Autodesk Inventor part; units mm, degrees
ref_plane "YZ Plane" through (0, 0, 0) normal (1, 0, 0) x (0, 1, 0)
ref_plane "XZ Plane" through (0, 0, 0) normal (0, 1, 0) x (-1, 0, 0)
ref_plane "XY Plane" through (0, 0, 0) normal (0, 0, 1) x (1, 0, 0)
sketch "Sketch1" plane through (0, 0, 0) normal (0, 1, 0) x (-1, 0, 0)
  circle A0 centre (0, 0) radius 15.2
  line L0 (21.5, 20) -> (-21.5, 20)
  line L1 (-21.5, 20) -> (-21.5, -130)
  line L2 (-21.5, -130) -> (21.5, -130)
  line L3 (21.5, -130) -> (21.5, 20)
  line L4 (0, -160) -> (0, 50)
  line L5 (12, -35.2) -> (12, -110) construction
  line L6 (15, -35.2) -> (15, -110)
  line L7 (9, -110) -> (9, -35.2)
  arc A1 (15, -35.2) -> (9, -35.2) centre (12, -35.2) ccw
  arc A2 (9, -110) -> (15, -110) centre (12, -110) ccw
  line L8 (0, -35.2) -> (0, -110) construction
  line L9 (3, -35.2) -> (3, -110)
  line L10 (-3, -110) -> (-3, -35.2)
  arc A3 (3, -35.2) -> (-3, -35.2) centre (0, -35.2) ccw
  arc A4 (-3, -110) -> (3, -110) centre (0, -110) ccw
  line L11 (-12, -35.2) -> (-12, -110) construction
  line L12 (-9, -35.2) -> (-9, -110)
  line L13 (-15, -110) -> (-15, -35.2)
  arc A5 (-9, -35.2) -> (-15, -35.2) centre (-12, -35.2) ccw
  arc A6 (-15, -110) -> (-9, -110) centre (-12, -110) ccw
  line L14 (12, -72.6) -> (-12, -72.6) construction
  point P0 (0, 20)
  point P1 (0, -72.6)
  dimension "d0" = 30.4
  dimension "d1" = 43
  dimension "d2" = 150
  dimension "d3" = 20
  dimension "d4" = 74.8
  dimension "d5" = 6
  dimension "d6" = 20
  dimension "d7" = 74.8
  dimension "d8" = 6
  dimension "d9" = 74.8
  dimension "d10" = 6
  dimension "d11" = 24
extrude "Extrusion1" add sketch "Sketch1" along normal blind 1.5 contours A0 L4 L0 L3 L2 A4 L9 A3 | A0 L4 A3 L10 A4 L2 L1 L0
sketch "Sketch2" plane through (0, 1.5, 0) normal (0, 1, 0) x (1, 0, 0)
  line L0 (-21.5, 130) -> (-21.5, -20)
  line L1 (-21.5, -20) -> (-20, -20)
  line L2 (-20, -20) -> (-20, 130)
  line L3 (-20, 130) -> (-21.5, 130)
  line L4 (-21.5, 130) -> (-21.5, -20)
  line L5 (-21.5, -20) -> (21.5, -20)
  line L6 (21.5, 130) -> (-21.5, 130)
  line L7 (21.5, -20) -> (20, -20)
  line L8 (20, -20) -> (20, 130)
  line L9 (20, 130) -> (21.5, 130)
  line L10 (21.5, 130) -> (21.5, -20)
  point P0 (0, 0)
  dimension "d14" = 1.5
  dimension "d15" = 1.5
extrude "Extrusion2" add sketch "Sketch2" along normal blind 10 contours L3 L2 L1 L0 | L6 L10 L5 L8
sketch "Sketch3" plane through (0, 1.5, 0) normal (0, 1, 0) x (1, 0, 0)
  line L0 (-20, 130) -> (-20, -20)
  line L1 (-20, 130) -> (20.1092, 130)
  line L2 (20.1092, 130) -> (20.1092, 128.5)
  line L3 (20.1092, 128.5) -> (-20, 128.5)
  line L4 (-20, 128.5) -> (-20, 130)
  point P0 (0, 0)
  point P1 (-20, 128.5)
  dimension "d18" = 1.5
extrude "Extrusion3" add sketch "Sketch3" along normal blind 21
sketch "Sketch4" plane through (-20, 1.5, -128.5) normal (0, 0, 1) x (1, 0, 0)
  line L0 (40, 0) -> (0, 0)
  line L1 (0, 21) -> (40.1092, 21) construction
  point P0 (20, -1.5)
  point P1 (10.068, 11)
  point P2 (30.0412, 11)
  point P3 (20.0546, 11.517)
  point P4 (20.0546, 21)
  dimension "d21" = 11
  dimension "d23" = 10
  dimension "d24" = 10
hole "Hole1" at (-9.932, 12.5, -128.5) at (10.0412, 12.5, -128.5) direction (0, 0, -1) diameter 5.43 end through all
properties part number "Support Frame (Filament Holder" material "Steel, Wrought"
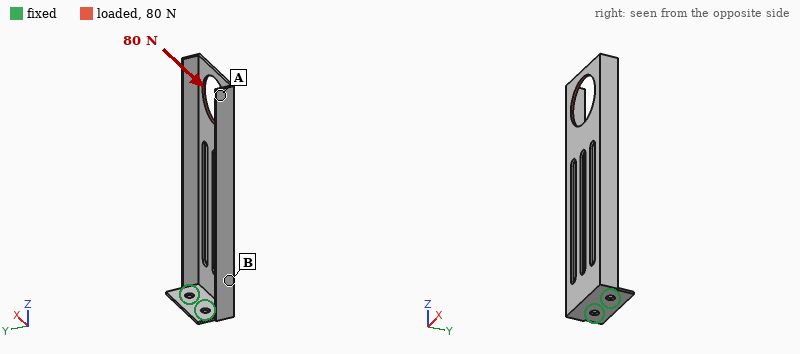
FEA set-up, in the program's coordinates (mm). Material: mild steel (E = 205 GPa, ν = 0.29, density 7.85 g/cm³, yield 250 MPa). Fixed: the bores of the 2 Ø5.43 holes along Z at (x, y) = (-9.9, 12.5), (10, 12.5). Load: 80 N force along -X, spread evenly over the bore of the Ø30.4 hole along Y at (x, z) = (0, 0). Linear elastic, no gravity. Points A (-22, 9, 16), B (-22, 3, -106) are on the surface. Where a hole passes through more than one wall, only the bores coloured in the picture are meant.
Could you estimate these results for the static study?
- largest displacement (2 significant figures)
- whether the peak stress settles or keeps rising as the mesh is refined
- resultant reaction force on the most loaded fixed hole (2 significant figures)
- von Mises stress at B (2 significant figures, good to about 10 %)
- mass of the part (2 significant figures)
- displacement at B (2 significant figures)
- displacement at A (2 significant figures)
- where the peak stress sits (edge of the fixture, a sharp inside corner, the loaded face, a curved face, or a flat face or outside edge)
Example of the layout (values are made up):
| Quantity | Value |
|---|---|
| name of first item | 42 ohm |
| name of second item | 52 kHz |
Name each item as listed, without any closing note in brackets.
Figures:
| Quantity | Value |
|---|---|
| largest displacement | 0.90 mm |
| whether the peak stress settles or keeps rising as the mesh is refined | keeps rising |
| resultant reaction force on the most loaded fixed hole | 370 N |
| von Mises stress at B | 39 MPa |
| mass of the part | 95 g |
| displacement at B | 0.14 mm |
| displacement at A | 0.84 mm |
| where the peak stress sits | edge of the fixture |
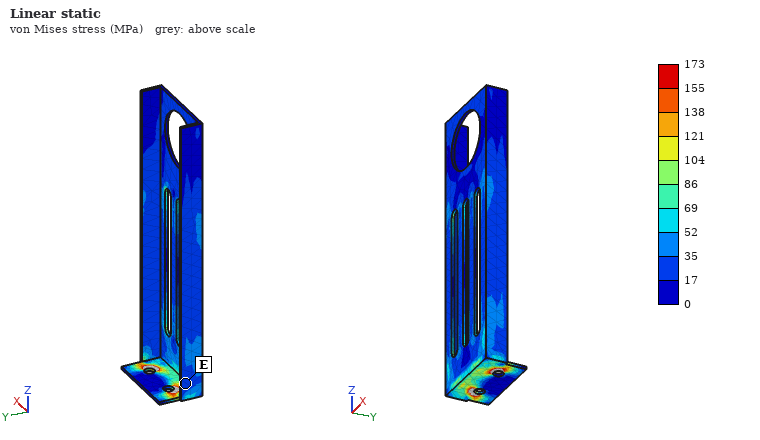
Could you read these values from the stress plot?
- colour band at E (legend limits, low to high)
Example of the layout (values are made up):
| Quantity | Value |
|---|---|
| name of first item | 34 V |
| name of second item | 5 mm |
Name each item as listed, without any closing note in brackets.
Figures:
| Quantity | Value |
|---|---|
| colour band at E | 17 to 35 MPa |
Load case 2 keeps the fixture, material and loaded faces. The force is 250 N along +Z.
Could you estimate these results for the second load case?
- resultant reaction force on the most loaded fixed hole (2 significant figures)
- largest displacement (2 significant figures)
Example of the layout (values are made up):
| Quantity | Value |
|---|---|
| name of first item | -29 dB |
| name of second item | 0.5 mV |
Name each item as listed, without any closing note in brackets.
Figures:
| Quantity | Value |
|---|---|
| resultant reaction force on the most loaded fixed hole | 130 N |
| largest displacement | 0.56 mm |
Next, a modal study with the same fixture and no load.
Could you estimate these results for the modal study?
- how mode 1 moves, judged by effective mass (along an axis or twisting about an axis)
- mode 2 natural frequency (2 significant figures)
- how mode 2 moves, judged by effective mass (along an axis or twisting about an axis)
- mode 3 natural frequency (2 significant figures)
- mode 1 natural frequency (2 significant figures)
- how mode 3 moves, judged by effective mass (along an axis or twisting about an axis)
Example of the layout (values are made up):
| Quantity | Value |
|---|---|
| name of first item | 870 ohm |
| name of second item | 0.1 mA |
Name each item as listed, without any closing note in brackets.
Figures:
| Quantity | Value |
|---|---|
| how mode 1 moves, judged by effective mass | along Y |
| mode 2 natural frequency | 240 Hz |
| how mode 2 moves, judged by effective mass | along X |
| mode 3 natural frequency | 480 Hz |
| mode 1 natural frequency | 130 Hz |
| how mode 3 moves, judged by effective mass | along X |
